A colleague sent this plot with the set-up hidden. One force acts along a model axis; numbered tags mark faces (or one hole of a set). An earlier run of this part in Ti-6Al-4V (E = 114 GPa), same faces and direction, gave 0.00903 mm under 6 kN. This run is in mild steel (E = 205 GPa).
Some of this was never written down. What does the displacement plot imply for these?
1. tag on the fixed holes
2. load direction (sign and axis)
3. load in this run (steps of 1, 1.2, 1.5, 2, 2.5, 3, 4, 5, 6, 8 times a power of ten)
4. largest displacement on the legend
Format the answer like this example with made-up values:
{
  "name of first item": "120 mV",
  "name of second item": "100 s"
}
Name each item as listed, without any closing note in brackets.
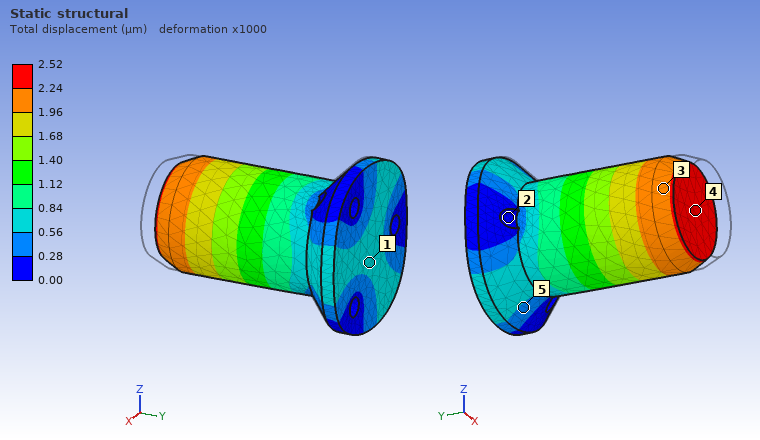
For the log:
{
  "tag on the fixed holes": "2",
  "load direction": "+Y",
  "load in this run": "3 kN",
  "largest displacement on the legend": "2.52 µm"
}
